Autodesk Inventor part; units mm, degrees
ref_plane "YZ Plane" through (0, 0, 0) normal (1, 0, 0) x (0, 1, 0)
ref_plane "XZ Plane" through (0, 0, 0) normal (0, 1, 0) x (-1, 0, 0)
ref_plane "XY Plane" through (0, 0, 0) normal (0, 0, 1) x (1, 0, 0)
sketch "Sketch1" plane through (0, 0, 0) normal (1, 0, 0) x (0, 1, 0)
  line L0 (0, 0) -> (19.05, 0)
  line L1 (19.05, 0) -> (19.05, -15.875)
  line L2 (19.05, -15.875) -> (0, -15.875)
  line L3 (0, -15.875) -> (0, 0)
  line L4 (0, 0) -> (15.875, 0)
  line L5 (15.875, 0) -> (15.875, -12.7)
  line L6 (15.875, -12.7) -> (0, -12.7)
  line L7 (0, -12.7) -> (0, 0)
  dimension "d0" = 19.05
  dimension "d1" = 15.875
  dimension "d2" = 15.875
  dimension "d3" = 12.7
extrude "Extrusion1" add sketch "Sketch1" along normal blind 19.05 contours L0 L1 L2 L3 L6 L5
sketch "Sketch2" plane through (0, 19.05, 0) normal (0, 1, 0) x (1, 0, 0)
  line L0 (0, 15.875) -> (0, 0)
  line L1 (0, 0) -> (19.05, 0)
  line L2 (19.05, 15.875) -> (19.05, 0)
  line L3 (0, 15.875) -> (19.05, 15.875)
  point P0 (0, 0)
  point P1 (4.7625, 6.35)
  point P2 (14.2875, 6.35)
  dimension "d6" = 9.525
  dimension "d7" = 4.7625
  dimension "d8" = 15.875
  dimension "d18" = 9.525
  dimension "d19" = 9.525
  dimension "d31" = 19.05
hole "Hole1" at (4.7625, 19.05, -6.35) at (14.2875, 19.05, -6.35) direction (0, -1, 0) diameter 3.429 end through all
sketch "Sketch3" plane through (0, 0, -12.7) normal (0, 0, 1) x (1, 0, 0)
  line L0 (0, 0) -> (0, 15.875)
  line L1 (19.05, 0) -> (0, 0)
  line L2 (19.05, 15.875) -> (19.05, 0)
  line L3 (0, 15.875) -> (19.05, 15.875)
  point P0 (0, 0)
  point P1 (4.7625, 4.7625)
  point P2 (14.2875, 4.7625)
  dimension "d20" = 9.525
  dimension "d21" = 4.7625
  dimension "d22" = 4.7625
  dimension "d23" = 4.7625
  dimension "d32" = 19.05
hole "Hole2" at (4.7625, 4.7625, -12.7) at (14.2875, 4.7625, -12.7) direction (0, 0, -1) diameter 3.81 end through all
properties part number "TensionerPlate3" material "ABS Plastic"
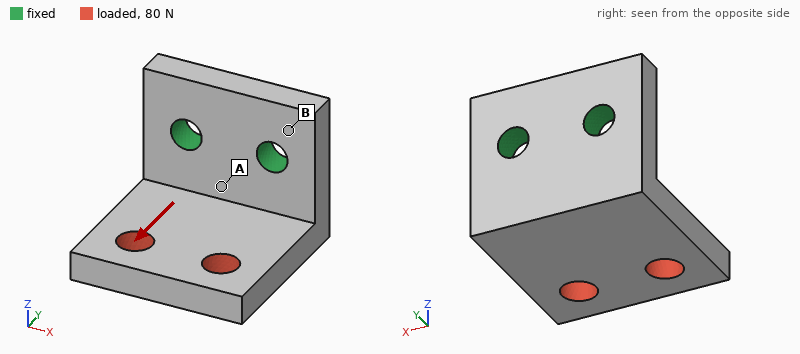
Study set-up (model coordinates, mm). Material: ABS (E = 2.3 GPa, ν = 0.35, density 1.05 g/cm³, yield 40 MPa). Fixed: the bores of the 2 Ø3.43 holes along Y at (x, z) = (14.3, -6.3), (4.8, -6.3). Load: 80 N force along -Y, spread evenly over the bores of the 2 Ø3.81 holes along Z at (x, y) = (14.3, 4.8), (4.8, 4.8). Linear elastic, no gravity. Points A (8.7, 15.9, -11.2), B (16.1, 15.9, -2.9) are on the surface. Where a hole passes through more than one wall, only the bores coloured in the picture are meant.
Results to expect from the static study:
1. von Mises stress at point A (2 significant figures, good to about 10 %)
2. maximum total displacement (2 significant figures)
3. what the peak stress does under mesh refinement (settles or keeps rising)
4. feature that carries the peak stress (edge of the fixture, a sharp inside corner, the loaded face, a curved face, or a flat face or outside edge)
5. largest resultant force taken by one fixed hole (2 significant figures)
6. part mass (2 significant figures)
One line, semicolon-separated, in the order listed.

6.5 MPa; 0.32 mm; keeps rising; edge of the fixture; 40 N; 1.9 g
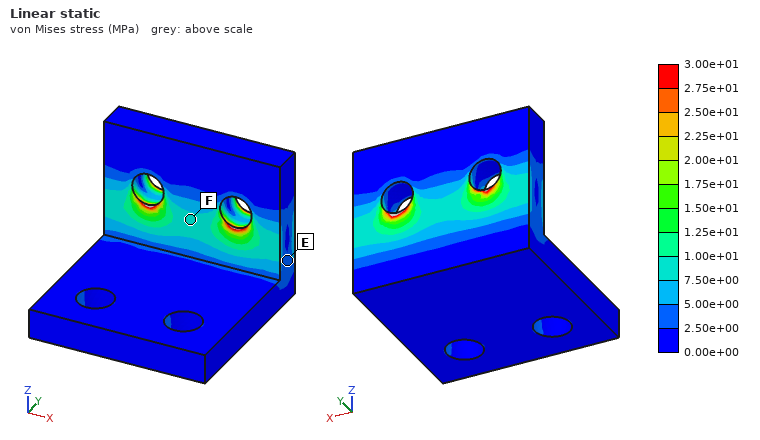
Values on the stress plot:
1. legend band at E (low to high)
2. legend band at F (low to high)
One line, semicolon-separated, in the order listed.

2.50e+00 to 5.00e+00 MPa; 7.50e+00 to 1.00e+01 MPa
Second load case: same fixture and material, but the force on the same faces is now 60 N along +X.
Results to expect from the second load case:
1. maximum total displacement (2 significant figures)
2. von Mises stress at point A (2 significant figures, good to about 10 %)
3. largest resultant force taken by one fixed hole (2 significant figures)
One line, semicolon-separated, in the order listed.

0.29 mm; 11 MPa; 75 N
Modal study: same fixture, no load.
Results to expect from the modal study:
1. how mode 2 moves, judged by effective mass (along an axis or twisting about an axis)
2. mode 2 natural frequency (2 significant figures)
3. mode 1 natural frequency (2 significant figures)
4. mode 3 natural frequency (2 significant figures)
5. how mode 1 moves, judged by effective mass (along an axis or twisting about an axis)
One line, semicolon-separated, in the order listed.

along X; 3200 Hz; 1700 Hz; 5000 Hz; along Z
